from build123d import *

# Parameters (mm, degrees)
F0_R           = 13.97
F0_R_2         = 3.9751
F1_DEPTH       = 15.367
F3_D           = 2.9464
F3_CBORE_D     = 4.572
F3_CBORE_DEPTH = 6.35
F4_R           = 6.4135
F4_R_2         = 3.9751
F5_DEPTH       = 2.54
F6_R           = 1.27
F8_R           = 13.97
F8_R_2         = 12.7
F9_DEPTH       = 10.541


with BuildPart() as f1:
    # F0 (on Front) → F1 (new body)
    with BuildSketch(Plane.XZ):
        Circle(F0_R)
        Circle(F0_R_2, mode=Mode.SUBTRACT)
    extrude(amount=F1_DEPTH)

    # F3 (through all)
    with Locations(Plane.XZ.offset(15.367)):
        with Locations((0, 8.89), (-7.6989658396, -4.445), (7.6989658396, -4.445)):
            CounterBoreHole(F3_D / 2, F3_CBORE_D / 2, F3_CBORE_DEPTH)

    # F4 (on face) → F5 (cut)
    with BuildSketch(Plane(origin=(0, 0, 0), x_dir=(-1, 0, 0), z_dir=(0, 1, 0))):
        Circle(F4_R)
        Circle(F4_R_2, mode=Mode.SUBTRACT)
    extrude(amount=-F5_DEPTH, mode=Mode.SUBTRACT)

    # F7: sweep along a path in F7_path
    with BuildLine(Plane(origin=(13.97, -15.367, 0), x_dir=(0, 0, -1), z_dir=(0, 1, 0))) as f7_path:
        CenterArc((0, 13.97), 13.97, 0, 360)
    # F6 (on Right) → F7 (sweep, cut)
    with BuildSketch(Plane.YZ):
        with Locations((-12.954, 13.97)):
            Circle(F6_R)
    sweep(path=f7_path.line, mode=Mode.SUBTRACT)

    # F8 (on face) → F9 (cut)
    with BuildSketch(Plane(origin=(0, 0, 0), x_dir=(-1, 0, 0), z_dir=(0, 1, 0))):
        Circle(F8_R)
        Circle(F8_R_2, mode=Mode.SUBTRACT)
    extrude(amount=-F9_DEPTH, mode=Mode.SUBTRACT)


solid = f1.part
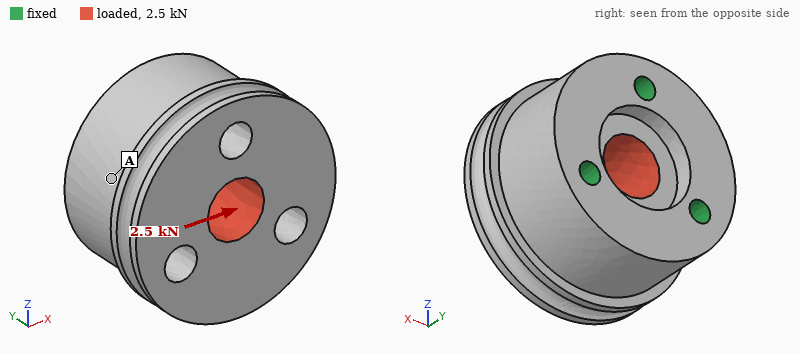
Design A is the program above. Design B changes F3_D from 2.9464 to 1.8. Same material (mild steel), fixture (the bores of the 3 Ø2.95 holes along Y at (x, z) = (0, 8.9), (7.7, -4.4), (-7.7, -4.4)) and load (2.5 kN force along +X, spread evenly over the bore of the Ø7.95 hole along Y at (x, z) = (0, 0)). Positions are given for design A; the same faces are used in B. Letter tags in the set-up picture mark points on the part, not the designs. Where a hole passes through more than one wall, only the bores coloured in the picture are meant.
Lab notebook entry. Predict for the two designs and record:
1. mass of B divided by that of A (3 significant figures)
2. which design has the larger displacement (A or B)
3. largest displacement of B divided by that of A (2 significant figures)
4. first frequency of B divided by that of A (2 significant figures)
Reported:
1.02
B
1.2
0.89
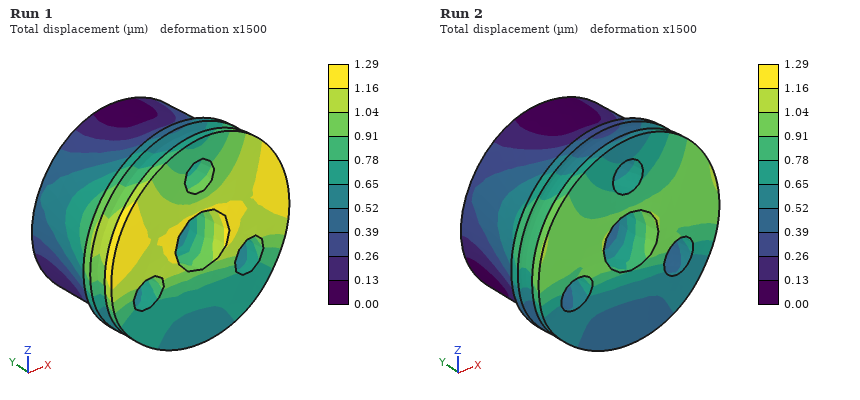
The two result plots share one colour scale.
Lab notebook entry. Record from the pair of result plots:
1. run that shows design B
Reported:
Run 1
